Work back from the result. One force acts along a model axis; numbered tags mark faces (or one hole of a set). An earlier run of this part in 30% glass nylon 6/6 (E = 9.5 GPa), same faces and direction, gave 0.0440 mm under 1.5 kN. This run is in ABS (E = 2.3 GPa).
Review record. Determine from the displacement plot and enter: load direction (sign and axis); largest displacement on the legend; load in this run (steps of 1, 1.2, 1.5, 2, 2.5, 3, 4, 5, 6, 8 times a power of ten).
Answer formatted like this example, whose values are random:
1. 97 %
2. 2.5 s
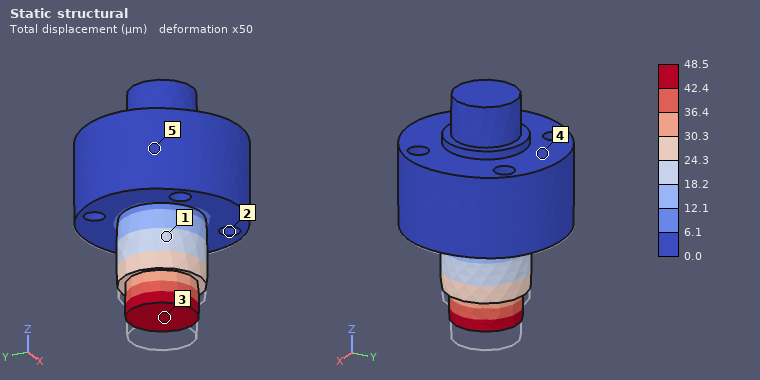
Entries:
1. +Z
2. 48.5 µm
3. 400 N
